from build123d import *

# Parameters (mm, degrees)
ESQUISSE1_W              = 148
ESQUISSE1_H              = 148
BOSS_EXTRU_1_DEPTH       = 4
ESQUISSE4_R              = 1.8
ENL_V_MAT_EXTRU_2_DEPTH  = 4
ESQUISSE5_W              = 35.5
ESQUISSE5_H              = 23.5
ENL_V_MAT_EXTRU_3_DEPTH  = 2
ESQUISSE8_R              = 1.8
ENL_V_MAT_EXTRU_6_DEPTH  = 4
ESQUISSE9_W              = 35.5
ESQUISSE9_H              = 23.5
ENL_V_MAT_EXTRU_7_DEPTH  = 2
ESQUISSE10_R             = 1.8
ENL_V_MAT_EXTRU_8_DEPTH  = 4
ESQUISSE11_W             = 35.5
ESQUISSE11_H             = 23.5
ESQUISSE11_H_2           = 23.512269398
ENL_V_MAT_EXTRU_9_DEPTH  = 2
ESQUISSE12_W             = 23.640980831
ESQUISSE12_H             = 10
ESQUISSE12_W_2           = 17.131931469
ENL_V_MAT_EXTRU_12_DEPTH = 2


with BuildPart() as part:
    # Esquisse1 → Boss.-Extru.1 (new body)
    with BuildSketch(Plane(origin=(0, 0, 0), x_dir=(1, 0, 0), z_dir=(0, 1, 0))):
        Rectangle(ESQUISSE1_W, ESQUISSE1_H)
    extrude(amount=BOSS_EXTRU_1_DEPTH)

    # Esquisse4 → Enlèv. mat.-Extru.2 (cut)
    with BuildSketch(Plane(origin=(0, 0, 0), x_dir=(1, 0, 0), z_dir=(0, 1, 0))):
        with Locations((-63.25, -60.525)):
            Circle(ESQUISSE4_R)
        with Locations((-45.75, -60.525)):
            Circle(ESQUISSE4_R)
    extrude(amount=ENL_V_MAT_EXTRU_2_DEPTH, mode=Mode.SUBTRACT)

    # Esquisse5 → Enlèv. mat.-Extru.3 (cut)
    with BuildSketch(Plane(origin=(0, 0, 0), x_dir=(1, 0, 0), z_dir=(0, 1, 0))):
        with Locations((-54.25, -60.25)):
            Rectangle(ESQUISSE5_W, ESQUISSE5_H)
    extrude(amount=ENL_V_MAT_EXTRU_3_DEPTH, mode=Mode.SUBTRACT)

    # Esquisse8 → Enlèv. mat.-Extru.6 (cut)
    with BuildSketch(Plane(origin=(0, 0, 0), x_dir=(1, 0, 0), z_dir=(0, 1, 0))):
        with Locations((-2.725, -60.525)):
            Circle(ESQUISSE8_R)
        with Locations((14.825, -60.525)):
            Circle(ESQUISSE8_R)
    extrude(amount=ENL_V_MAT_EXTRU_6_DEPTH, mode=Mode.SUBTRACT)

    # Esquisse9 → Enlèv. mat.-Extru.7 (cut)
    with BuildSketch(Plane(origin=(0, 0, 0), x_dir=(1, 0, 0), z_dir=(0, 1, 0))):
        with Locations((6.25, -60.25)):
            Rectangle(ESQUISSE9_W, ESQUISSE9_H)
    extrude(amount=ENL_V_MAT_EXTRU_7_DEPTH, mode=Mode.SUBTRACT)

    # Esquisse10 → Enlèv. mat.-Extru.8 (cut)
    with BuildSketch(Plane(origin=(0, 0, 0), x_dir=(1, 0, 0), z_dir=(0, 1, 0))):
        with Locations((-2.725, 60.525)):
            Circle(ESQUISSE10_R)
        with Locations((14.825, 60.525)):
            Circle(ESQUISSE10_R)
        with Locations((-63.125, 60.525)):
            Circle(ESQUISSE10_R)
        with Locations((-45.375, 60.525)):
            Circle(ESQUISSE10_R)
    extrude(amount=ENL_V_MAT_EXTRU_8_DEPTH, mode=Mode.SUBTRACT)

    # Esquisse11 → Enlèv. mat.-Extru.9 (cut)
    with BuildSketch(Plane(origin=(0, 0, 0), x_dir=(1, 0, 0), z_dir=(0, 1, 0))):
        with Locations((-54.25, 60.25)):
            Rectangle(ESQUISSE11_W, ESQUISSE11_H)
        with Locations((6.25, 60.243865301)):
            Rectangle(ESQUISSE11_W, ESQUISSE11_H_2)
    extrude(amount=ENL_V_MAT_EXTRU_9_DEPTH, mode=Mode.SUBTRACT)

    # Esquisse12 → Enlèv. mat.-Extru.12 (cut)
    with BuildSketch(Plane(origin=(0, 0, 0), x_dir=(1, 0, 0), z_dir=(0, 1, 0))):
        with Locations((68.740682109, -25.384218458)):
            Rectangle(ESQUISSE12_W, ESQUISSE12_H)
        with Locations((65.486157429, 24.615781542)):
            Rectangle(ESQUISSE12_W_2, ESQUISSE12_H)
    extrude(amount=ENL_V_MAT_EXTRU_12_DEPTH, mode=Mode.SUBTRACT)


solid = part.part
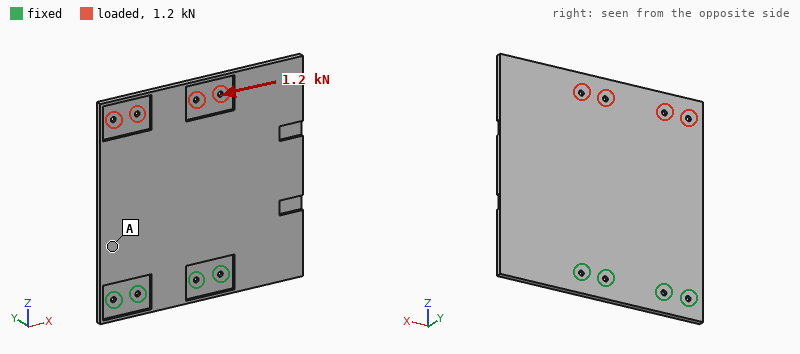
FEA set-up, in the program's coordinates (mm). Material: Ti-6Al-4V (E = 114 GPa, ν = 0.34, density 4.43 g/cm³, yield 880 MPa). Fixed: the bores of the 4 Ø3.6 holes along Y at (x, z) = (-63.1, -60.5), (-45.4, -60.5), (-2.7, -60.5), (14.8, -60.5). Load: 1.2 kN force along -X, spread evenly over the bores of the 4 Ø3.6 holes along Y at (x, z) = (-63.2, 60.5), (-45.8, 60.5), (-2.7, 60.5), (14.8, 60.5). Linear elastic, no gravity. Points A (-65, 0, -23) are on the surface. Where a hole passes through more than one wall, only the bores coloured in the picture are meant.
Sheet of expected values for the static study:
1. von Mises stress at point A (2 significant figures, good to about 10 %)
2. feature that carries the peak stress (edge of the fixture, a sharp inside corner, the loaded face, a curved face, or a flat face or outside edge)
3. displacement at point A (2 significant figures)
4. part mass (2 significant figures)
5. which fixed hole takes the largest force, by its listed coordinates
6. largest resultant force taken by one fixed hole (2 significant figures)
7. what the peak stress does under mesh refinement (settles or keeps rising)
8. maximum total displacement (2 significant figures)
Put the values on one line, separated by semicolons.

6.4 MPa; edge of the fixture; 0.051 mm; 350 g; (14.8, -60.5); 1.7 kN; keeps rising; 0.21 mm
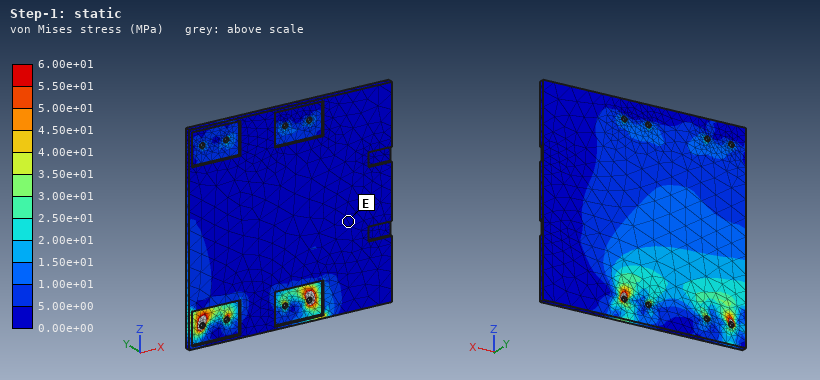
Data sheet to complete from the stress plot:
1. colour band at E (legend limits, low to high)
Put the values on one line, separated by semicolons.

0.00e+00 to 5.00e+00 MPa
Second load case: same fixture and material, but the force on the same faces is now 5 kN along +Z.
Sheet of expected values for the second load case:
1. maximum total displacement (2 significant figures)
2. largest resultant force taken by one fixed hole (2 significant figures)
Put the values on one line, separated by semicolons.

0.46 mm; 1.3 kN
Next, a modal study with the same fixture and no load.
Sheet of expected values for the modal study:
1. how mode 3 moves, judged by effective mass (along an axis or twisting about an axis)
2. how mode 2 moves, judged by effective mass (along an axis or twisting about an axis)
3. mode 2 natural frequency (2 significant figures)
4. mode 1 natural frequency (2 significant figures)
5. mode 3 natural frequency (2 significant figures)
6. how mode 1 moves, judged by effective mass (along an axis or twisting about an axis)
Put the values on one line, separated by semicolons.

along Y; twisting about Z; 300 Hz; 120 Hz; 690 Hz; along Y
